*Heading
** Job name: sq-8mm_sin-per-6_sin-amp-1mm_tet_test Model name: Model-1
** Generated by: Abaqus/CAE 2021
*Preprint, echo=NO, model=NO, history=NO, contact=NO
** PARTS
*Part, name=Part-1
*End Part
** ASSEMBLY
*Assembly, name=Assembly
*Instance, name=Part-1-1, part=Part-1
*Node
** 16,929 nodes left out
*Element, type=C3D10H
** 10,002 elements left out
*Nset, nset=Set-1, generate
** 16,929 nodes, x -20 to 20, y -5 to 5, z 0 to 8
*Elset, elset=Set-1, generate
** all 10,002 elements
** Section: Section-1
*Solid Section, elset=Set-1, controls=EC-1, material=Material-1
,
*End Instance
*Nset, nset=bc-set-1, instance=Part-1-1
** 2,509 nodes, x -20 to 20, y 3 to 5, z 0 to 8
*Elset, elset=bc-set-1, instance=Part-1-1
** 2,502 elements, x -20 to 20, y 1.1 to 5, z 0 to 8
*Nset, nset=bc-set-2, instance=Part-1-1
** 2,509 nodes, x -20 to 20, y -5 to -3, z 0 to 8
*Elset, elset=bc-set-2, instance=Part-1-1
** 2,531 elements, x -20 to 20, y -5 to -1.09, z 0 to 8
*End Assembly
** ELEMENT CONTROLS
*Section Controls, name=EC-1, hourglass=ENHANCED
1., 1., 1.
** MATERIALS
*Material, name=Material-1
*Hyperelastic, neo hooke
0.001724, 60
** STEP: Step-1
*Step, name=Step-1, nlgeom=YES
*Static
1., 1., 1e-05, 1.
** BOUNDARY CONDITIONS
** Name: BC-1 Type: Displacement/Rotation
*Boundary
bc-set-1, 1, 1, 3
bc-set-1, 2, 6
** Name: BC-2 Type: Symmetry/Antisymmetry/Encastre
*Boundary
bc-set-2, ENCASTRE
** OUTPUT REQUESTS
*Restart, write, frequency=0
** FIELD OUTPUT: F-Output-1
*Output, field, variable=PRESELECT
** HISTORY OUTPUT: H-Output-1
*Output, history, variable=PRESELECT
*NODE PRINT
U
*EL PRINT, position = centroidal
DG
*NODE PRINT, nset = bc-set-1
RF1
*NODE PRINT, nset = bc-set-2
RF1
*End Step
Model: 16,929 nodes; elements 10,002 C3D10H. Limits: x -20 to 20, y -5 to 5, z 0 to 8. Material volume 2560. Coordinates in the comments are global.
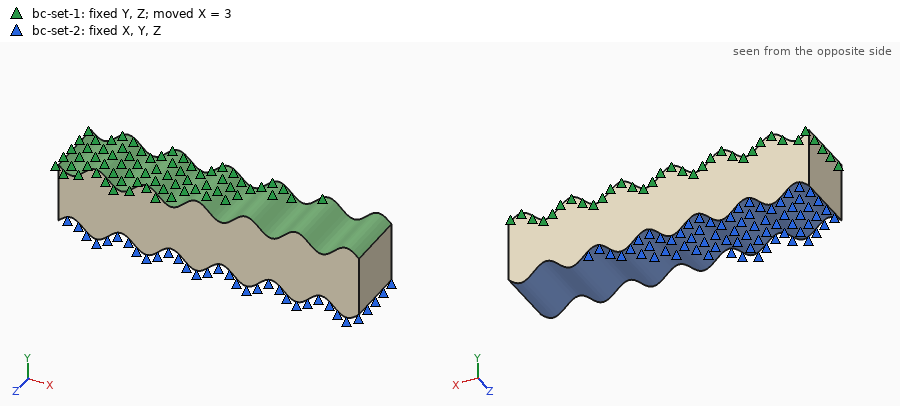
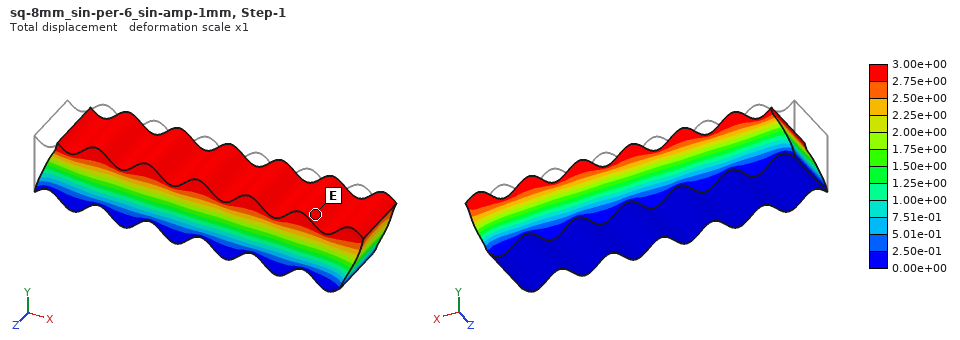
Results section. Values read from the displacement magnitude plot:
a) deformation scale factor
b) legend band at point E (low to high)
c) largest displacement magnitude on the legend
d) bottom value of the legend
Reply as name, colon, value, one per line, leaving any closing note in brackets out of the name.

deformation scale factor: 1
legend band at point E: 2.75e+00 to 3.00e+00
largest displacement magnitude on the legend: 3.00e+00
bottom value of the legend: 0.00e+00
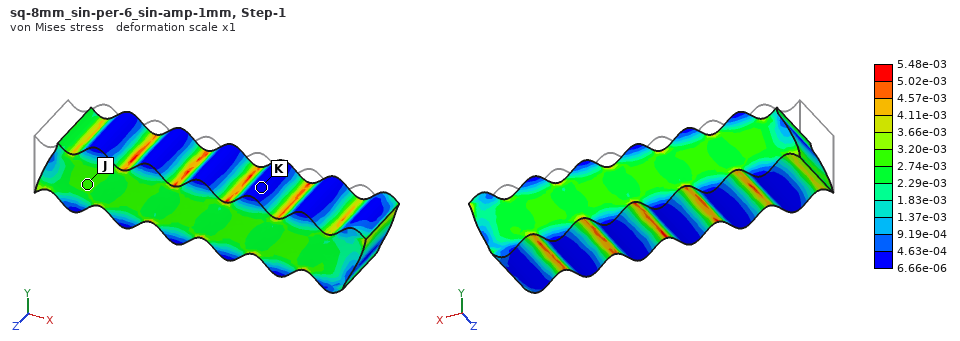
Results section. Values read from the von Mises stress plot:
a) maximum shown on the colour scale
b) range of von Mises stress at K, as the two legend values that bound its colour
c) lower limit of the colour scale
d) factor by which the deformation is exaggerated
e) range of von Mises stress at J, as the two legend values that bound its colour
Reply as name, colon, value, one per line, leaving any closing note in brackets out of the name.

maximum shown on the colour scale: 5.48e-03
range of von Mises stress at K, as the two legend values that bound its colour: 6.66e-06 to 4.63e-04
lower limit of the colour scale: 6.66e-06
factor by which the deformation is exaggerated: 1
range of von Mises stress at J, as the two legend values that bound its colour: 2.74e-03 to 3.20e-03
